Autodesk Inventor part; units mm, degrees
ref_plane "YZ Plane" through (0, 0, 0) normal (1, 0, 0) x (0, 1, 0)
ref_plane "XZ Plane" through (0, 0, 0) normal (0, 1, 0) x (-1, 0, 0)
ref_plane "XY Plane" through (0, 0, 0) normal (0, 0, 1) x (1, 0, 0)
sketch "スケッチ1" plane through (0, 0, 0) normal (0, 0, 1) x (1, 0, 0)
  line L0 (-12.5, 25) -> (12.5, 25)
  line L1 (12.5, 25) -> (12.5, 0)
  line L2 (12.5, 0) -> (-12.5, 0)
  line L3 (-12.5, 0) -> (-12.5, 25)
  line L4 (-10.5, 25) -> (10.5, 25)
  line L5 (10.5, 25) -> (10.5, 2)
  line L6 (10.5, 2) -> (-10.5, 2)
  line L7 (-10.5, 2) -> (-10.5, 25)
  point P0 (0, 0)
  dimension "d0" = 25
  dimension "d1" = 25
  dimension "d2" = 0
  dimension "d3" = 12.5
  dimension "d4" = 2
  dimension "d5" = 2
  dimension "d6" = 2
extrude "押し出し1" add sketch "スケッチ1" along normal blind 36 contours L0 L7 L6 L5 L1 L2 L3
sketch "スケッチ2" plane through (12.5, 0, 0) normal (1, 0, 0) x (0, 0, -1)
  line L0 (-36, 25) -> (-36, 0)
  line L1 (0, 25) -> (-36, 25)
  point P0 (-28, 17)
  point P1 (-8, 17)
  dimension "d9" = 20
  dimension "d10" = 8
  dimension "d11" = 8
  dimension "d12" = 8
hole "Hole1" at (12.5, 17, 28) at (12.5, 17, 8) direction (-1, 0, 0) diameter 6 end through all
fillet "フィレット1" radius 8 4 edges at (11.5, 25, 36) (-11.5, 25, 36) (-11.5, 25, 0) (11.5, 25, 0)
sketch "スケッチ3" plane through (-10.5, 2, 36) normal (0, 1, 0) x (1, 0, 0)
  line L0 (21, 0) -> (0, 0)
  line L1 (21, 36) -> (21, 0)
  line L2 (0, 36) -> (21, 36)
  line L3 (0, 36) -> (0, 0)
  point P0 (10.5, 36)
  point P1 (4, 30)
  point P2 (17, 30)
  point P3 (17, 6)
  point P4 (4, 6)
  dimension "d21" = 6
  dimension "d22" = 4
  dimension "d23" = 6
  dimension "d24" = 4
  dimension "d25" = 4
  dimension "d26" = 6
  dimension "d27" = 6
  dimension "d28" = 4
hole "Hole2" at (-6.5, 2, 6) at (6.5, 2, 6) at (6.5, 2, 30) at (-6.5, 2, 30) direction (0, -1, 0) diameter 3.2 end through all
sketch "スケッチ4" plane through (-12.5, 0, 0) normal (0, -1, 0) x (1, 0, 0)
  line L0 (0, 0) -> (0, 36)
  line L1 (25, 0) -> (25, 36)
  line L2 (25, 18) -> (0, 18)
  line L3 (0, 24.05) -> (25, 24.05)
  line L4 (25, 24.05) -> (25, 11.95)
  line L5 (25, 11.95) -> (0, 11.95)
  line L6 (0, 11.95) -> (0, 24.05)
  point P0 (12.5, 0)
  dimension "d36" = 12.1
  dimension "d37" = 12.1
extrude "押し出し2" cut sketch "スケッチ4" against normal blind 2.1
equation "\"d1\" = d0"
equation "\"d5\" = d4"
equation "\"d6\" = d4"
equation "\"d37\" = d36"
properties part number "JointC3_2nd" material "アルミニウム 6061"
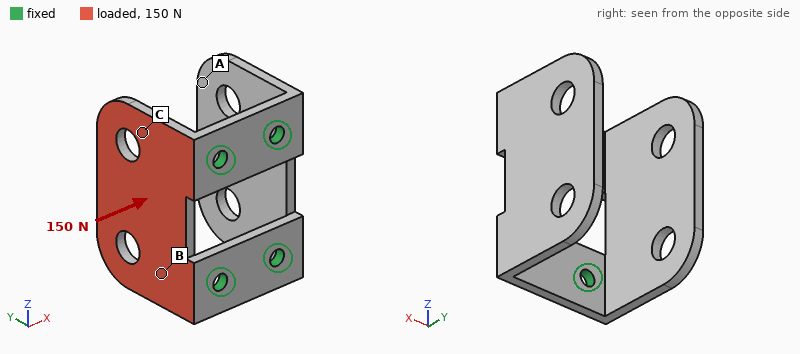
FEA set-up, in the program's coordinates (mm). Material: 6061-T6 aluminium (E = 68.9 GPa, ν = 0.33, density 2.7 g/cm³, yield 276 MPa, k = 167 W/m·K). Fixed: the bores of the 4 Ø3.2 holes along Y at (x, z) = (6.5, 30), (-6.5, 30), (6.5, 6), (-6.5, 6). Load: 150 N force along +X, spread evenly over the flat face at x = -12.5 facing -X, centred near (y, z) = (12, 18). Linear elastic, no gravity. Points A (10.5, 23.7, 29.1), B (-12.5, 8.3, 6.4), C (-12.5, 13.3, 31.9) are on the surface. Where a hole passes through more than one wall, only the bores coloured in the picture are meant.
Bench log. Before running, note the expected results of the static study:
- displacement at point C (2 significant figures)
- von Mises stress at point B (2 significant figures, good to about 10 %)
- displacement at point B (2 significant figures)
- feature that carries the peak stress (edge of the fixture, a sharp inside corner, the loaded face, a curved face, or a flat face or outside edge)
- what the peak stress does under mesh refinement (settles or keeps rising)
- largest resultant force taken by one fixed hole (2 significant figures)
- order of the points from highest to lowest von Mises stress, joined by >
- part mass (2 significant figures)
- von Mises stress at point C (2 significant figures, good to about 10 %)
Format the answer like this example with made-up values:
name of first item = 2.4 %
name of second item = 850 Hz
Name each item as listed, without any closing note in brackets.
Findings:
displacement at point C = 0.13 mm
von Mises stress at point B = 35 MPa
displacement at point B = 0.073 mm
feature that carries the peak stress = a sharp inside corner
what the peak stress does under mesh refinement = keeps rising
largest resultant force taken by one fixed hole = 71 N
order of the points from highest to lowest von Mises stress, joined by > = B > C > A
part mass = 11 g
von Mises stress at point C = 21 MPa
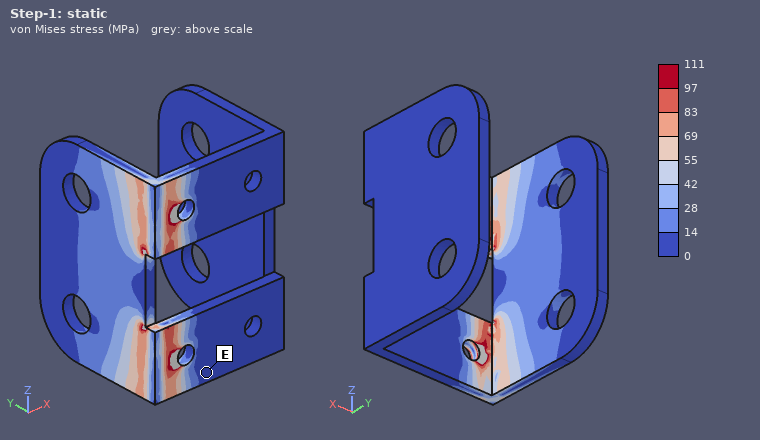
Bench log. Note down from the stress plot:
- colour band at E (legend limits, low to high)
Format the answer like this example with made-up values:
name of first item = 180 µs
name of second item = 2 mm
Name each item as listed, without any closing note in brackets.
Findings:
colour band at E = 0 to 14 MPa
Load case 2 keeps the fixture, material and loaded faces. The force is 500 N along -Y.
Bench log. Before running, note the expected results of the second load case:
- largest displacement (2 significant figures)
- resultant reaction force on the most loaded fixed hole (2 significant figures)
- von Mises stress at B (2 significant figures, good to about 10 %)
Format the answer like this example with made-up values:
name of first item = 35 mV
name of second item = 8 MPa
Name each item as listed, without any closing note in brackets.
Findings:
largest displacement = 0.22 mm
resultant reaction force on the most loaded fixed hole = 270 N
von Mises stress at B = 22 MPa
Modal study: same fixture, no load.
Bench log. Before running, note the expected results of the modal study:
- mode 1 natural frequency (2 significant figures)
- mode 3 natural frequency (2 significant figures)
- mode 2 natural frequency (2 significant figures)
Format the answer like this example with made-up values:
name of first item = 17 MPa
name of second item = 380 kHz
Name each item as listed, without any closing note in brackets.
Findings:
mode 1 natural frequency = 2100 Hz
mode 3 natural frequency = 5000 Hz
mode 2 natural frequency = 2100 Hz
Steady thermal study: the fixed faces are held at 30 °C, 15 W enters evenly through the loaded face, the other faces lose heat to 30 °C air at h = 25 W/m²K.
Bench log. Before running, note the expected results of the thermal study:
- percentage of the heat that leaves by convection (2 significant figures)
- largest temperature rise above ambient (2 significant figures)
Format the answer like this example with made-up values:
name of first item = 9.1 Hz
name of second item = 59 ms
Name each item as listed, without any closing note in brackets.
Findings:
percentage of the heat that leaves by convection = 3.7 %
largest temperature rise above ambient = 26 K
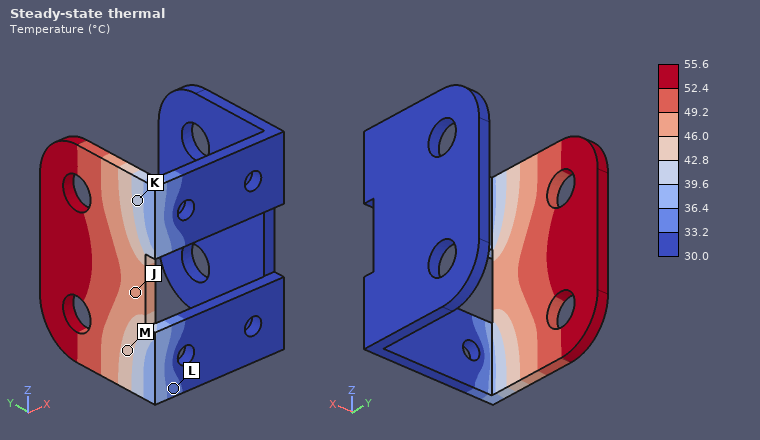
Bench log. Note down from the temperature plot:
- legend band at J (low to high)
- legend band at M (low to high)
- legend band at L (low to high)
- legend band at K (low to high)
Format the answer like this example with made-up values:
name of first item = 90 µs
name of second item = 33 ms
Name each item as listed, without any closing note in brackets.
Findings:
legend band at J = 46.0 to 49.2 °C
legend band at M = 42.8 to 46.0 °C
legend band at L = 33.2 to 36.4 °C
legend band at K = 39.6 to 42.8 °C
